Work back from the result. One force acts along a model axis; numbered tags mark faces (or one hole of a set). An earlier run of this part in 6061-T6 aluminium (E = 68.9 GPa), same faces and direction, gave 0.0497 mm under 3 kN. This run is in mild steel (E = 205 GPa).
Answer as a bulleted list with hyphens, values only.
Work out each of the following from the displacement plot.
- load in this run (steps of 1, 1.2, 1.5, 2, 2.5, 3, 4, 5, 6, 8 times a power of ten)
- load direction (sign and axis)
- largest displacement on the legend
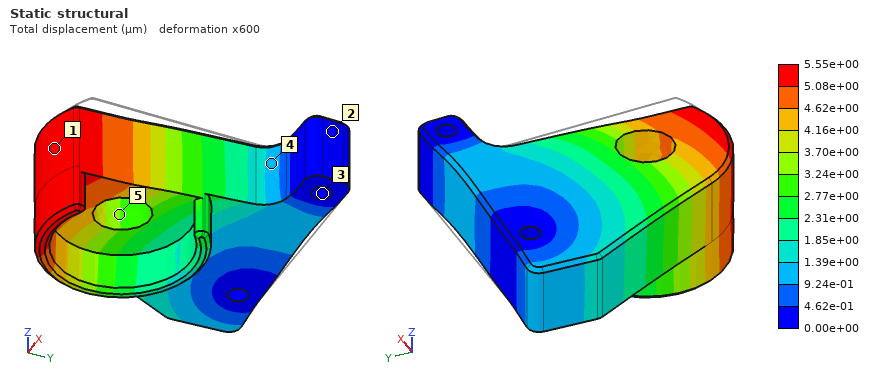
- 1 kN
- -X
- 5.55e+00 µm
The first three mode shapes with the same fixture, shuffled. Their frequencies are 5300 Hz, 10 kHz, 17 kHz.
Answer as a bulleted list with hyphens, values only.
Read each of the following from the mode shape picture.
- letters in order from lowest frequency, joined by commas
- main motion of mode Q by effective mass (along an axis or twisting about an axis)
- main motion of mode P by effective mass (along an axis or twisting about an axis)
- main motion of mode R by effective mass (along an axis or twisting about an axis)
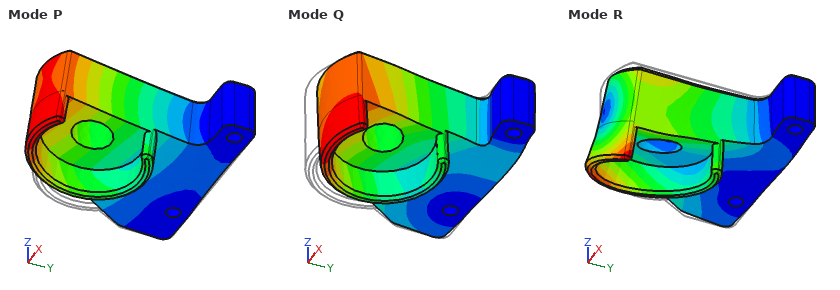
- P, Q, R
- along X
- along Z
- twisting about Y
